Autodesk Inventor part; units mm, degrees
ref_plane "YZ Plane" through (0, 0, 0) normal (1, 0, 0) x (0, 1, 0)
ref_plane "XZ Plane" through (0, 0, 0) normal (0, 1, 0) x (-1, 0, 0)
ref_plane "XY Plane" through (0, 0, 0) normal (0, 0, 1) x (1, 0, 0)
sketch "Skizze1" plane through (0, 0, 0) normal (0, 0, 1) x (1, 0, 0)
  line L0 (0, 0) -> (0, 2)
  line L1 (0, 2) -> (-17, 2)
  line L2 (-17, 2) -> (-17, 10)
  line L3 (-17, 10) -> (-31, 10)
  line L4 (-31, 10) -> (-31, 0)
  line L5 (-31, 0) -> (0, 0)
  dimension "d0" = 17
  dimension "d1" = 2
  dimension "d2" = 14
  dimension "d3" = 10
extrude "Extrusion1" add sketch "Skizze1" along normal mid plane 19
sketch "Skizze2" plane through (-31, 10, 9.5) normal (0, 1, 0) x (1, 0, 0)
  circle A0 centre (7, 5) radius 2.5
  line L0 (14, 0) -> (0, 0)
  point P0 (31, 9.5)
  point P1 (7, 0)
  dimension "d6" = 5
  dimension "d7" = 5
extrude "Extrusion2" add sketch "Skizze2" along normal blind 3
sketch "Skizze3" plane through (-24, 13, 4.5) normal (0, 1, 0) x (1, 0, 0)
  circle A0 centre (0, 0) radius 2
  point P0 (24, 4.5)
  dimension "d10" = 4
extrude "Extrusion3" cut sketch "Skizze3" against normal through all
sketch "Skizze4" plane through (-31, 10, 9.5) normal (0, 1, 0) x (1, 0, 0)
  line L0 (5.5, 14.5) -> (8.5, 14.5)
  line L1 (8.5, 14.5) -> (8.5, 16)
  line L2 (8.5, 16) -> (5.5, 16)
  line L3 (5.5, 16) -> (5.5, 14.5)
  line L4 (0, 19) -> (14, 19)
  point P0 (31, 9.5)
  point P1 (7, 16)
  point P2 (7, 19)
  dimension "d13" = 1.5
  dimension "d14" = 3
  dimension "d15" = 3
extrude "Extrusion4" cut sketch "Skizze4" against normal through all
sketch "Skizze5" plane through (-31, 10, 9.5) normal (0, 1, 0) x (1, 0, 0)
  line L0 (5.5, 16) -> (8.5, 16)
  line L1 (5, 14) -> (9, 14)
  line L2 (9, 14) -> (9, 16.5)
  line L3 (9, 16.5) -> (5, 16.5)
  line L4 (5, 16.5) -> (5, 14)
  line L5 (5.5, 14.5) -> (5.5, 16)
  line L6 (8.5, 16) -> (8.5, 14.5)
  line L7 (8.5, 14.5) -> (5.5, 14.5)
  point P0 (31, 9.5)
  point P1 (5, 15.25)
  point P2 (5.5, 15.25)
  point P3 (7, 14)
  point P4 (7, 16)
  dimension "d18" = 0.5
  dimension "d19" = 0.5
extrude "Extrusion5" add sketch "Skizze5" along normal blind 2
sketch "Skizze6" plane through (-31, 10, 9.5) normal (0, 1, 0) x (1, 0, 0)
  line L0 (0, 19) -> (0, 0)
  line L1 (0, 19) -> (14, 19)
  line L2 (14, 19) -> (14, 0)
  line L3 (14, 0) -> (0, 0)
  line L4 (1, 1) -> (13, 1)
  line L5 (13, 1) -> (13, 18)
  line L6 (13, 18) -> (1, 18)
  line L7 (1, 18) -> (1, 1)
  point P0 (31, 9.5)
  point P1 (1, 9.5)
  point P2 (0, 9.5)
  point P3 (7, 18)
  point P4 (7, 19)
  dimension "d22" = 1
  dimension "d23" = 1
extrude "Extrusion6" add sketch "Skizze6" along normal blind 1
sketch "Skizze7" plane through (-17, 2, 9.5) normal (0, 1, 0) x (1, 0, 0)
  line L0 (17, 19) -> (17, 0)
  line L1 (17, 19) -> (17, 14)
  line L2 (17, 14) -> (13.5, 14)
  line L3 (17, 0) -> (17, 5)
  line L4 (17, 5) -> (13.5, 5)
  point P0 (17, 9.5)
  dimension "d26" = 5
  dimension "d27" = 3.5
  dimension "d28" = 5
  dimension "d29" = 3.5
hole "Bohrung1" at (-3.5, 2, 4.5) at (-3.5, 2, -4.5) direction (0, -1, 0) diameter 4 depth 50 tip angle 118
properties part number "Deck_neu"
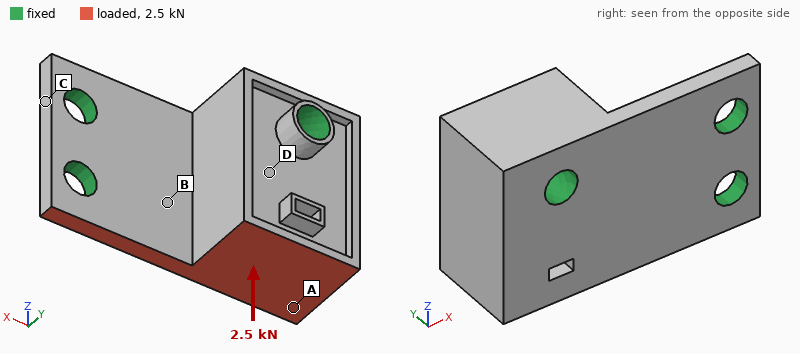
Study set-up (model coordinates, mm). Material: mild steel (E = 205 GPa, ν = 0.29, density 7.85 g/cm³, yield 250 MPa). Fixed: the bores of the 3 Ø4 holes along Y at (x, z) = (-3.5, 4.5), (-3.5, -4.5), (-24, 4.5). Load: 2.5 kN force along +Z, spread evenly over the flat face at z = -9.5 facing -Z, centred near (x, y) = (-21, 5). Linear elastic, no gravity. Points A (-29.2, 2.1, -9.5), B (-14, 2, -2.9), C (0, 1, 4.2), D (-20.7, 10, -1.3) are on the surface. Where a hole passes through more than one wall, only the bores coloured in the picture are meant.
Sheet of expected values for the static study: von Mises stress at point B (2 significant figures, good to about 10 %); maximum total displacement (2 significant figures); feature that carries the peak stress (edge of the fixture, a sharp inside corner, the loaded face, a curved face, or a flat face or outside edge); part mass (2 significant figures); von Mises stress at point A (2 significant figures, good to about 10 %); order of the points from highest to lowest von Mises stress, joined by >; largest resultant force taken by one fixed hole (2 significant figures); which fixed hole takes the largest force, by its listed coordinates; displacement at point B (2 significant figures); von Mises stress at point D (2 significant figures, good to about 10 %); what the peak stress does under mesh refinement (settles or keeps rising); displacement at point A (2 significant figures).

8.8 MPa
2.6 µm
a sharp inside corner
25 g
14 MPa
D > A > B > C
2.1 kN
(-24, 4.5)
0.65 µm
21 MPa
keeps rising
1.1 µm
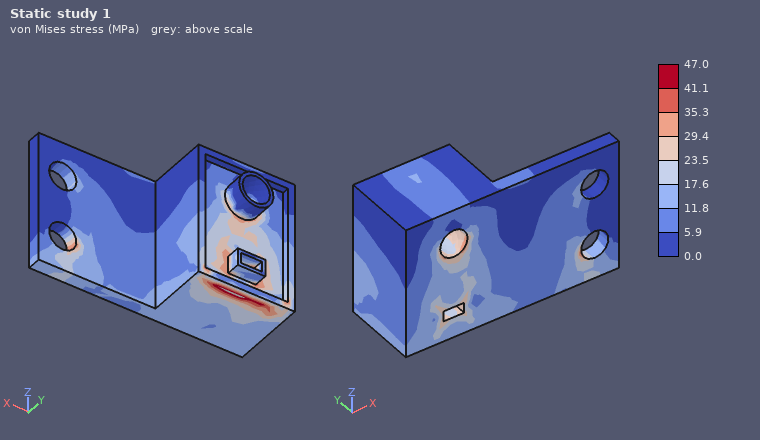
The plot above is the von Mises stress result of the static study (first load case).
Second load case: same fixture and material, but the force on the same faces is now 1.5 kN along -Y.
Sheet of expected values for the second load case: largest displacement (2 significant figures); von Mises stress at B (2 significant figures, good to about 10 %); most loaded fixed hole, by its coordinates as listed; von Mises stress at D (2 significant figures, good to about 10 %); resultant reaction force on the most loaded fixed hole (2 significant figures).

9.4 µm
19 MPa
(-24, 4.5)
47 MPa
1.3 kN
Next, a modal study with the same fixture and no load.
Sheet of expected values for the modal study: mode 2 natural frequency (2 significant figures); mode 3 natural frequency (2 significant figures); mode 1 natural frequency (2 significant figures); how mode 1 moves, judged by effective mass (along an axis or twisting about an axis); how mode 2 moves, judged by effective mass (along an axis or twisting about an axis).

34 kHz
46 kHz
31 kHz
along Y
along X
